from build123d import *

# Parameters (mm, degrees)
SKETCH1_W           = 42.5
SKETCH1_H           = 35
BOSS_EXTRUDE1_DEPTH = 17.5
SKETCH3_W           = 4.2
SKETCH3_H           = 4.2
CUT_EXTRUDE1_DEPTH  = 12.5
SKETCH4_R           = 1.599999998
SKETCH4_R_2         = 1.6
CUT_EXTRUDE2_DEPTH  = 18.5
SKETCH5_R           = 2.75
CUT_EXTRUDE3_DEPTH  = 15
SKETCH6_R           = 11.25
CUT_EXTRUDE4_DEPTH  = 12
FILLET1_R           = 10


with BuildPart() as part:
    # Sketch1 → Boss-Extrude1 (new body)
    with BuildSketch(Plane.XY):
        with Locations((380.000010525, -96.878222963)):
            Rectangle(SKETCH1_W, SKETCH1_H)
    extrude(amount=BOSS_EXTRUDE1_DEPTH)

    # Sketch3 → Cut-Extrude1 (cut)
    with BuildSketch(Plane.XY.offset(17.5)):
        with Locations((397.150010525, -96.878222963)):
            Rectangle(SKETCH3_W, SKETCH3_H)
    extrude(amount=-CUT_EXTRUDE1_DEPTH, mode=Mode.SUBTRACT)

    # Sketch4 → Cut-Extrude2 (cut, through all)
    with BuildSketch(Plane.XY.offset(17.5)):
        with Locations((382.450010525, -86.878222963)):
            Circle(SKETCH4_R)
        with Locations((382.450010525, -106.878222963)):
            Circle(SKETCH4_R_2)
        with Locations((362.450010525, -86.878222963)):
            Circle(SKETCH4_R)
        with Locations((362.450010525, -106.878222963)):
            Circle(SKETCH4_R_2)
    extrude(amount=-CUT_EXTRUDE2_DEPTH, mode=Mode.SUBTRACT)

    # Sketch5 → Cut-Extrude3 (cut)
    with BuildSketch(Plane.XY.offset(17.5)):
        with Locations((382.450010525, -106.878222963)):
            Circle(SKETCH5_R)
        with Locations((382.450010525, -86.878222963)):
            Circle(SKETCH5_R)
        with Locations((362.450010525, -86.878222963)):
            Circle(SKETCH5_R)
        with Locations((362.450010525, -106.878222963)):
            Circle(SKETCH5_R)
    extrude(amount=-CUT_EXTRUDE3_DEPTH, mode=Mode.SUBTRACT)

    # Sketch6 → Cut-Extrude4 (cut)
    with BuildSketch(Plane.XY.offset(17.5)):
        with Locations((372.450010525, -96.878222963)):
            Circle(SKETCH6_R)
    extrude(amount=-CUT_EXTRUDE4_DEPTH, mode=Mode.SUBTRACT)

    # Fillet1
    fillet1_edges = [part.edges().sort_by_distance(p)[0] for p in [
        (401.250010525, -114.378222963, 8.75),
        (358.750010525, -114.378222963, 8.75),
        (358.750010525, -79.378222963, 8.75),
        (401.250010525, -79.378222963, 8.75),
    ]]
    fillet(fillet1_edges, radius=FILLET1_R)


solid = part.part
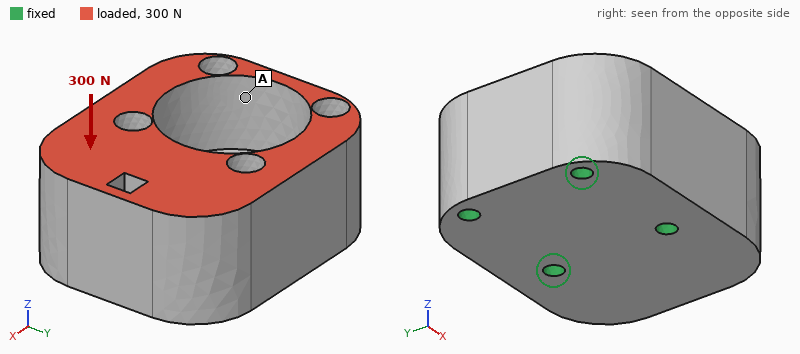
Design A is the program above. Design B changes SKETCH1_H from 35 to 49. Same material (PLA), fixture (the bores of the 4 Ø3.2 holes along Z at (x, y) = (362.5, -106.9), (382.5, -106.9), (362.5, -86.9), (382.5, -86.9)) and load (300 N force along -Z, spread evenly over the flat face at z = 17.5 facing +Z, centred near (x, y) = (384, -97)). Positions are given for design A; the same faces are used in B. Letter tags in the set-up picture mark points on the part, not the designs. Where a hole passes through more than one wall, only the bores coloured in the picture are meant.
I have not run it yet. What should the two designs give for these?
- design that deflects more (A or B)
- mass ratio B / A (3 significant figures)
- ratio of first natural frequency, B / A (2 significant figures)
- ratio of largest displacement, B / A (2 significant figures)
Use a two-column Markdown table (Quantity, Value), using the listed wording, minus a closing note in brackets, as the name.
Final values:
| Quantity | Value |
|---|---|
| design that deflects more | A |
| mass ratio B / A | 1.58 |
| ratio of first natural frequency, B / A | 0.87 |
| ratio of largest displacement, B / A | 0.72 |
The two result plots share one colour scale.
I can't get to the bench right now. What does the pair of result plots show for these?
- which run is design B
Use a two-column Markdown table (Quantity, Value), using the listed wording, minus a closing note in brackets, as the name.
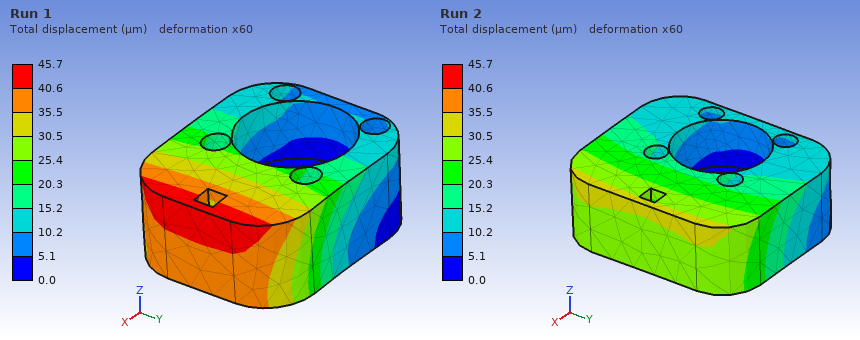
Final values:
| Quantity | Value |
|---|---|
| which run is design B | Run 2 |
